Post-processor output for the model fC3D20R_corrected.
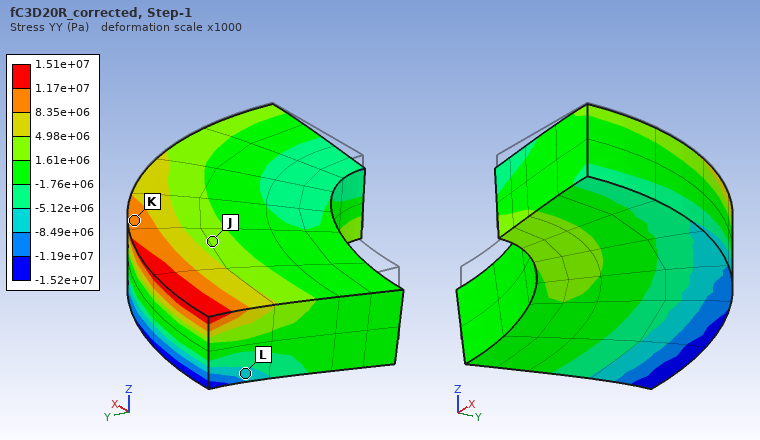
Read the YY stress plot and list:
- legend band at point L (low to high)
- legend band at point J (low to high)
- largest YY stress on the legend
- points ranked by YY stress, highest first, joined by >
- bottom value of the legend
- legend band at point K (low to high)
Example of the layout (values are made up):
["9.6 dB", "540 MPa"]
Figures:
["-8.49e+06 to -5.12e+06 Pa", "1.61e+06 to 4.98e+06 Pa", "1.51e+07 Pa", "K > J > L", "-1.52e+07 Pa", "8.35e+06 to 1.17e+07 Pa"]
